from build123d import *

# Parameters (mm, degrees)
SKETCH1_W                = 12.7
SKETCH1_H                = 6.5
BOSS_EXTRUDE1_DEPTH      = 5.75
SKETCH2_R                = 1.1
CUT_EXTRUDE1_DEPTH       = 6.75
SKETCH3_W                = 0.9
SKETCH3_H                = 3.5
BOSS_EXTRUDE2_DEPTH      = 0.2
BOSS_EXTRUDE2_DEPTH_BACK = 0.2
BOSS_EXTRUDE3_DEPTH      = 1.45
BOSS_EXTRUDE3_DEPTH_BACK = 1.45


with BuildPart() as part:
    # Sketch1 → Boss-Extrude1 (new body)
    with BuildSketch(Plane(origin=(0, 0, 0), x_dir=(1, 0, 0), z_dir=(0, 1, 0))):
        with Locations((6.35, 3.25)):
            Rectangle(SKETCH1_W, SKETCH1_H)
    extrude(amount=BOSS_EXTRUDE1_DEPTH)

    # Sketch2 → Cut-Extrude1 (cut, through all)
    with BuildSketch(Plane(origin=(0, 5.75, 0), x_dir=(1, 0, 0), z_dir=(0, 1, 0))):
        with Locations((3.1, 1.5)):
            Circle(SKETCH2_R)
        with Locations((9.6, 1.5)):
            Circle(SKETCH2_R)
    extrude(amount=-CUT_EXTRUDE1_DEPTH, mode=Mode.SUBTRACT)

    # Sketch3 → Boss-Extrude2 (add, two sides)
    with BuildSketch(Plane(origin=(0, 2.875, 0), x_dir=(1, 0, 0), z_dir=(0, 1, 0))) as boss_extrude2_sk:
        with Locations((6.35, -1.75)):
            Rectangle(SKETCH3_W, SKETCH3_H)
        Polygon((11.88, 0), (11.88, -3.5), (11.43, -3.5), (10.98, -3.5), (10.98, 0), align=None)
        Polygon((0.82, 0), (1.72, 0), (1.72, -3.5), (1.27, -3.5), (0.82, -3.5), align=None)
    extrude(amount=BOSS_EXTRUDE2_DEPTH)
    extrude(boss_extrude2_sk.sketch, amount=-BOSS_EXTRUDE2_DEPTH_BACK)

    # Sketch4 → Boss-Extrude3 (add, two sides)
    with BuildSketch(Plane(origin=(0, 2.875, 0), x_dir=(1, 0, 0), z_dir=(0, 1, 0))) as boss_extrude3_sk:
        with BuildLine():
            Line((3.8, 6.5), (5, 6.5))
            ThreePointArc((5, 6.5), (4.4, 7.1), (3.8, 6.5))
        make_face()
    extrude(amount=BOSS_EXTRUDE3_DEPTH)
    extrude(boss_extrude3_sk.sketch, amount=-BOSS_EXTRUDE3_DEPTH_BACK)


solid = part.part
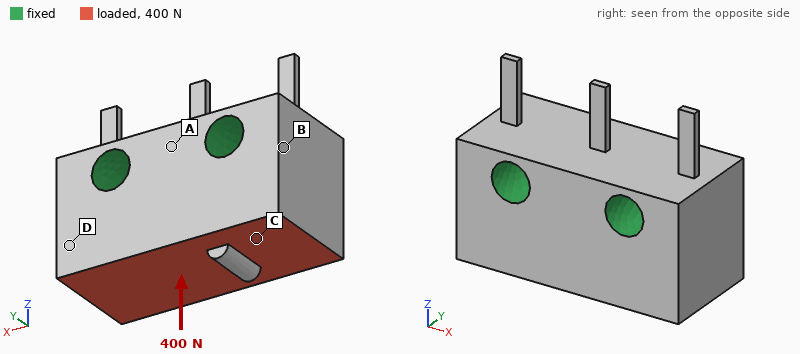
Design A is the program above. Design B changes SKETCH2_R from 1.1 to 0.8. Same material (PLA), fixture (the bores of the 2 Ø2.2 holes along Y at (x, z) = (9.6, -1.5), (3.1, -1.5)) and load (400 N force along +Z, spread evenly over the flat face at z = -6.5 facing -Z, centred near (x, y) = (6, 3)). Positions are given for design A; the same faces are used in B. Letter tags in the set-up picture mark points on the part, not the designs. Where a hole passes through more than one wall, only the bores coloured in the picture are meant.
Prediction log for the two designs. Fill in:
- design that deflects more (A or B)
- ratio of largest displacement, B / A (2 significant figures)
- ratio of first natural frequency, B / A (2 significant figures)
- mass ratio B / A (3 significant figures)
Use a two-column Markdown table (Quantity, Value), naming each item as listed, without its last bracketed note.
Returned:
| Quantity | Value |
|---|---|
| design that deflects more | B |
| ratio of largest displacement, B / A | 1.1 |
| ratio of first natural frequency, B / A | 1.00 |
| mass ratio B / A | 1.05 |
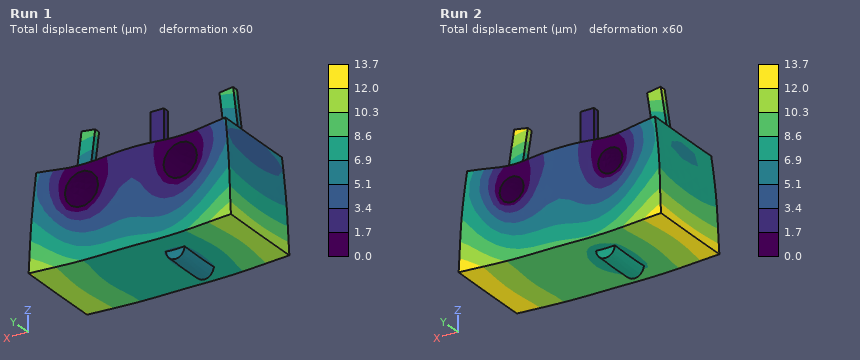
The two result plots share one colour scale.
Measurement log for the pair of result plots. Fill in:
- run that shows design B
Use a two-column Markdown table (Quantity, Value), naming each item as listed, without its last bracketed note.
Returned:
| Quantity | Value |
|---|---|
| run that shows design B | Run 2 |
